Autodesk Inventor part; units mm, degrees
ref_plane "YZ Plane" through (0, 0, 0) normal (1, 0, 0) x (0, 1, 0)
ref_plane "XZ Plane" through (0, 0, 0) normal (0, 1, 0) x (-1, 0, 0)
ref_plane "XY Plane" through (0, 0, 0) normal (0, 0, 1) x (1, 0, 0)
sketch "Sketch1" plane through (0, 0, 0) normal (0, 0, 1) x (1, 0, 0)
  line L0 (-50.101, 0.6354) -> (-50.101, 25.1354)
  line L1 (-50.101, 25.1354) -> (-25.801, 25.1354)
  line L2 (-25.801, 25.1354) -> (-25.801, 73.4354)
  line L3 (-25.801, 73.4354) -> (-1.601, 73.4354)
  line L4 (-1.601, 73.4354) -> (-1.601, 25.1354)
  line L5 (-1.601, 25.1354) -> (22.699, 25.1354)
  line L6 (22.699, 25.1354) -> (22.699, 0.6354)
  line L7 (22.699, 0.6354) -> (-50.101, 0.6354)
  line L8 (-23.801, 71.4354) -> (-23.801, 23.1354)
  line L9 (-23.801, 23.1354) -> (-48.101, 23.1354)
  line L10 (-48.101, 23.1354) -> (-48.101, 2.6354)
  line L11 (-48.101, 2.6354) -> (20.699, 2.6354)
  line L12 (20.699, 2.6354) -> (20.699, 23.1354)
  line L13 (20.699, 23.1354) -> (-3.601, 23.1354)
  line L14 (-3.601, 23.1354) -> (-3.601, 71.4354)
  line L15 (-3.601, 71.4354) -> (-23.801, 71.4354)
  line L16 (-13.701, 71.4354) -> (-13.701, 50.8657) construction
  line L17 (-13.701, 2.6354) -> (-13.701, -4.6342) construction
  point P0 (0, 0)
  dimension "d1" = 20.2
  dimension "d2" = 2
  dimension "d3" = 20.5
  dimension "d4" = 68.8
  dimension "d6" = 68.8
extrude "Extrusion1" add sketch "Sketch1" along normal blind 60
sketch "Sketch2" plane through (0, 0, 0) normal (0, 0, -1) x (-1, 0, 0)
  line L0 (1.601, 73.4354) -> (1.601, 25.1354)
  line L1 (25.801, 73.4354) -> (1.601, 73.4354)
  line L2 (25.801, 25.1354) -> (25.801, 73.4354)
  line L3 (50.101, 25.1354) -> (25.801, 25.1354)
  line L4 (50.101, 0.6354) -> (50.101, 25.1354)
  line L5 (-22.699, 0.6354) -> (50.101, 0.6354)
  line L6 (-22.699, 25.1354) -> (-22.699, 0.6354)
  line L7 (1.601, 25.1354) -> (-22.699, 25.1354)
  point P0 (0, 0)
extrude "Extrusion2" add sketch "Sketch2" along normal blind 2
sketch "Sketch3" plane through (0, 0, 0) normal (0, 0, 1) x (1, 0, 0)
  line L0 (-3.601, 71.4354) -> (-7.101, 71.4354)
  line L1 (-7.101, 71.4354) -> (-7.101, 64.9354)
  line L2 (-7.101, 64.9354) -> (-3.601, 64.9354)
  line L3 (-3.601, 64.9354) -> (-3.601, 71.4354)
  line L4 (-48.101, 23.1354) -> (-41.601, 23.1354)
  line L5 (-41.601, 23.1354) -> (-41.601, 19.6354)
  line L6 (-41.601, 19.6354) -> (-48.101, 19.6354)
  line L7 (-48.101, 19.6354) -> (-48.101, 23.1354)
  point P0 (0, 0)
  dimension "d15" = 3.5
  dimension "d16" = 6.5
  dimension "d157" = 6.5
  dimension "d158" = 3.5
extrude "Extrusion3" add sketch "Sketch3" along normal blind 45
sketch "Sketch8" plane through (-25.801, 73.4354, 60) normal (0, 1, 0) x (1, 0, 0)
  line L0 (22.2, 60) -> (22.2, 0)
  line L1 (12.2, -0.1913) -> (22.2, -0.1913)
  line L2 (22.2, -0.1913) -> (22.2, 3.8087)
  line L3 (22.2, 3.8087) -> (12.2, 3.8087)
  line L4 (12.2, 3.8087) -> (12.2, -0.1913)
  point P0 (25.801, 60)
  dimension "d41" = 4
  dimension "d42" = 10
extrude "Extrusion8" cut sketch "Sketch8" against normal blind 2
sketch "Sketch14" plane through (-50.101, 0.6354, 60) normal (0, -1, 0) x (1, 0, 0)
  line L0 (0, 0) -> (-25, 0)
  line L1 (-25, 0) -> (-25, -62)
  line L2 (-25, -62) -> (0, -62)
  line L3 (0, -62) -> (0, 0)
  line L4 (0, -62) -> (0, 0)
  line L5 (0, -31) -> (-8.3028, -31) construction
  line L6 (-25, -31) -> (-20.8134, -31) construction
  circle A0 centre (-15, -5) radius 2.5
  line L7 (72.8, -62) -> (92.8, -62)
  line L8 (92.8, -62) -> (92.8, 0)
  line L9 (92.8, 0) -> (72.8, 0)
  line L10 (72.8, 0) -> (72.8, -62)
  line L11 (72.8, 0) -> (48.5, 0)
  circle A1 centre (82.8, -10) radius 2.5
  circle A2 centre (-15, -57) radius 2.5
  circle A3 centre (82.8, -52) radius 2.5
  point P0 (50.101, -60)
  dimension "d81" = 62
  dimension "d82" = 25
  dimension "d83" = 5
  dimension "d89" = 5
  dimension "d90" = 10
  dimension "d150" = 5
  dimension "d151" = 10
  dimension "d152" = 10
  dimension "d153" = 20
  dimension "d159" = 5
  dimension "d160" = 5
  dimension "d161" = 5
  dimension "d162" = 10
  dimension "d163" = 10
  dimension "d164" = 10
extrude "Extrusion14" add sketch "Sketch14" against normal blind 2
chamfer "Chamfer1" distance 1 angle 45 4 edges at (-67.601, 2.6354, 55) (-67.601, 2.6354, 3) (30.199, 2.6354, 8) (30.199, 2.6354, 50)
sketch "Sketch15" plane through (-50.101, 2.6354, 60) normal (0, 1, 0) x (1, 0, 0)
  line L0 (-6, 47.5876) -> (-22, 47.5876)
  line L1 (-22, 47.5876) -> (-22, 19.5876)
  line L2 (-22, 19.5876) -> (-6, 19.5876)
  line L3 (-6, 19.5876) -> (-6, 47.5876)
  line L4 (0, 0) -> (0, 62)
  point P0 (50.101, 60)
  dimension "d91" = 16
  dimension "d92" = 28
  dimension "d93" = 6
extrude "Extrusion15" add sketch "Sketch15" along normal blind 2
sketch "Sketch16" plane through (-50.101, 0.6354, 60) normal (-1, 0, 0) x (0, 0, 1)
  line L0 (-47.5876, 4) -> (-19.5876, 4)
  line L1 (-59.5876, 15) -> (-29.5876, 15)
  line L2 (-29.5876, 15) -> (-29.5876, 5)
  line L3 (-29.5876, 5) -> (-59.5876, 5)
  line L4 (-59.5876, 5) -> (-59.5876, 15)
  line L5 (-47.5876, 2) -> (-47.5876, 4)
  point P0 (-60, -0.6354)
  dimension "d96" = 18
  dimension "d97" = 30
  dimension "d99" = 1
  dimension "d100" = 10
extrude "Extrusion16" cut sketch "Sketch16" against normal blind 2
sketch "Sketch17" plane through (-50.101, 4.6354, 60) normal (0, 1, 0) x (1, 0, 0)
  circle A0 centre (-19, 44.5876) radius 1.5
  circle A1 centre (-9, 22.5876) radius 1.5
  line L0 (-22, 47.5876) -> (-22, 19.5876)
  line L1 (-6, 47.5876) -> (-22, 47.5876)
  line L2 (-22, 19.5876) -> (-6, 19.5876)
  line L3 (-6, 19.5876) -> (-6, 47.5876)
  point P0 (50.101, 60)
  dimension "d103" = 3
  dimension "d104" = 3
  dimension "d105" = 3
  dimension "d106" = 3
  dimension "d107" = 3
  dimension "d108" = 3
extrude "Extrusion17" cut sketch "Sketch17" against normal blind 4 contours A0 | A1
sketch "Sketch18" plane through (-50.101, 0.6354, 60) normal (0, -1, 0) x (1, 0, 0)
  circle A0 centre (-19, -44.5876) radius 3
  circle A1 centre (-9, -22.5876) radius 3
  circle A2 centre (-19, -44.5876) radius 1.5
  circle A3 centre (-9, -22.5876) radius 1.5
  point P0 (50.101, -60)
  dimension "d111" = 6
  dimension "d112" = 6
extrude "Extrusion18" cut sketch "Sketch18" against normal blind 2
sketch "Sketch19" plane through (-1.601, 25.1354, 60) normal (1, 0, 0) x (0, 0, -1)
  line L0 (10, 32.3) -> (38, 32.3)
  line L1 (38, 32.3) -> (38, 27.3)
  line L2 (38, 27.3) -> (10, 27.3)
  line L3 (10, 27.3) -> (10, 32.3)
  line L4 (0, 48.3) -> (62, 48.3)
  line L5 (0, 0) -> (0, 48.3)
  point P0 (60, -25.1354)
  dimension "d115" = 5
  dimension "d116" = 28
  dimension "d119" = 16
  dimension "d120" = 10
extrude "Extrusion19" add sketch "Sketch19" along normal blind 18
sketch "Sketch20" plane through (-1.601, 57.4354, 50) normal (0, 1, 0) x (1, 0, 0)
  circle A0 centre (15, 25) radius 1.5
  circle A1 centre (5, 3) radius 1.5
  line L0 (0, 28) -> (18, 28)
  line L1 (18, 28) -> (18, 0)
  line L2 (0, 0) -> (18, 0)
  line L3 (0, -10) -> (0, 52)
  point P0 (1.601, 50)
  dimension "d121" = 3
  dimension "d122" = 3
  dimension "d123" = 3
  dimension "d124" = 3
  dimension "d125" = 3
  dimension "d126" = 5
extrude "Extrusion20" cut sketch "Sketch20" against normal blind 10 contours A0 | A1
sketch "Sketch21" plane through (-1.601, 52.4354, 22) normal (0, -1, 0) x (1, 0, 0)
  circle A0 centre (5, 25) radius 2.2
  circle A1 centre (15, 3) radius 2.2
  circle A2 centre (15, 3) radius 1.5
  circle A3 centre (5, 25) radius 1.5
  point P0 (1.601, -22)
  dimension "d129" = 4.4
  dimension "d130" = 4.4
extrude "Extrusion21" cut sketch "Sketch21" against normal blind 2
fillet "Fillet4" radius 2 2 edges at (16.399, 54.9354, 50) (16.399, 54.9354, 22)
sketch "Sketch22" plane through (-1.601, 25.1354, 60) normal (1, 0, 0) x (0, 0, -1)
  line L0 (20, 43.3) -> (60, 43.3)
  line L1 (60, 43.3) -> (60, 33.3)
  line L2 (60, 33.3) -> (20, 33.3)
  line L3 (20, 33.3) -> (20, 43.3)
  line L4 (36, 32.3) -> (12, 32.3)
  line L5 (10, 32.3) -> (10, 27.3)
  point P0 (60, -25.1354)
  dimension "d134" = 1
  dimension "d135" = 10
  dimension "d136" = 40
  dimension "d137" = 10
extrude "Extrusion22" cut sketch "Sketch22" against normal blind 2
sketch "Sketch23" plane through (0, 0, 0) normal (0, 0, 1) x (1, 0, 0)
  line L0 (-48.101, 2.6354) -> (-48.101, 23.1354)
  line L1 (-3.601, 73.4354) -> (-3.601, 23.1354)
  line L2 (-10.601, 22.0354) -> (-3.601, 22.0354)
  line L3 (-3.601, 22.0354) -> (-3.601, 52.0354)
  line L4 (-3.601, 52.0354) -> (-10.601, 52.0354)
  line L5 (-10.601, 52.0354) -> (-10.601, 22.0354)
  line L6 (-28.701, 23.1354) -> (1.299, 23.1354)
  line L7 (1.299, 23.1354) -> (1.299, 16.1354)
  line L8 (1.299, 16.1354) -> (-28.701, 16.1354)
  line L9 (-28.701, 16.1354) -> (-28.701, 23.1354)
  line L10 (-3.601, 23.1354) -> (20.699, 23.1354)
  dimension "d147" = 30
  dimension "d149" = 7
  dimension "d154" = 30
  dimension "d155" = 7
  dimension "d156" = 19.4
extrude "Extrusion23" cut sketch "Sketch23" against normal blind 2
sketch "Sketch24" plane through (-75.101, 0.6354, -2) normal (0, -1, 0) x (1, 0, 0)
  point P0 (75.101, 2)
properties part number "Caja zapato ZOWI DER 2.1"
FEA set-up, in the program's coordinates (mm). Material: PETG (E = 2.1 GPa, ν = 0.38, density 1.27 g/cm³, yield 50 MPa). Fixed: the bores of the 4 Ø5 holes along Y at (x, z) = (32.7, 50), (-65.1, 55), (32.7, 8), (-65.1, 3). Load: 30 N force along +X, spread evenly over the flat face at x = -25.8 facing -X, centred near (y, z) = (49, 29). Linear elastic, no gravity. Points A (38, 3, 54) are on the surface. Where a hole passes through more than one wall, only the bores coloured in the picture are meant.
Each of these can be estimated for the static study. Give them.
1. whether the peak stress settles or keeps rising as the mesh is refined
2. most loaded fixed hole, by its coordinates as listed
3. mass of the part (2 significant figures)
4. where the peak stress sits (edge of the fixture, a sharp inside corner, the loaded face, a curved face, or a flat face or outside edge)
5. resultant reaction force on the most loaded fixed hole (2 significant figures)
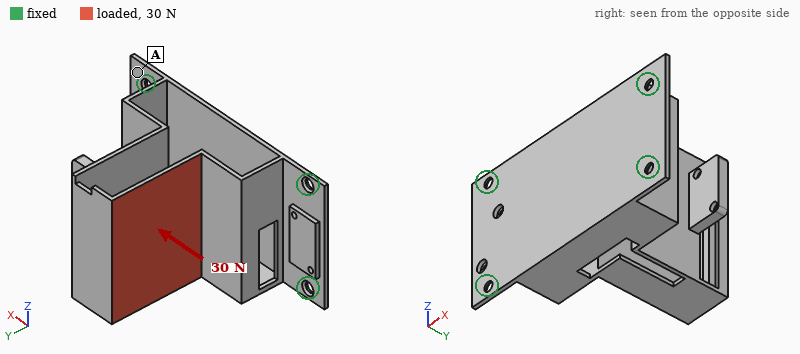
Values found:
keeps rising
(32.7, 8)
61 g
edge of the fixture
18 N
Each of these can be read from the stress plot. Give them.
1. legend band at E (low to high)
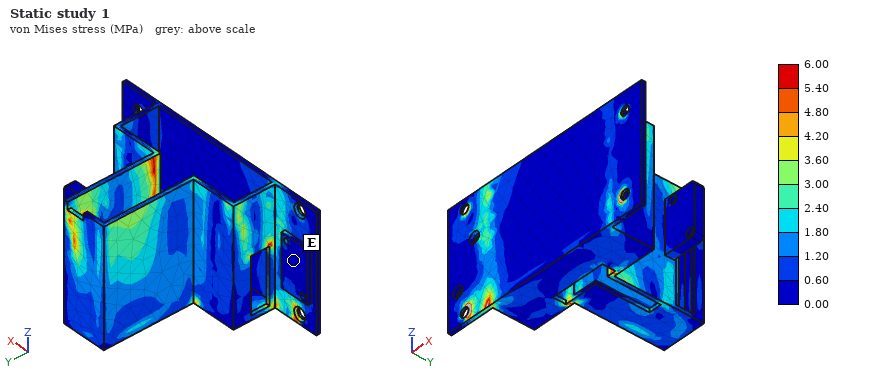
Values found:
0.00 to 0.60 MPa
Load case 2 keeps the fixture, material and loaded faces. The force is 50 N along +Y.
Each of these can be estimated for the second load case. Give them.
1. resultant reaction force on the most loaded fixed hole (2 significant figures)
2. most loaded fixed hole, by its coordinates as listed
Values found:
36 N
(-65.1, 3)
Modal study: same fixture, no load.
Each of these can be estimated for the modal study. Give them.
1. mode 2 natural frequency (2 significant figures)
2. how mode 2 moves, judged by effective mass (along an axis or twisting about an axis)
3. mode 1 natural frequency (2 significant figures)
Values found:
190 Hz
along X
160 Hz
